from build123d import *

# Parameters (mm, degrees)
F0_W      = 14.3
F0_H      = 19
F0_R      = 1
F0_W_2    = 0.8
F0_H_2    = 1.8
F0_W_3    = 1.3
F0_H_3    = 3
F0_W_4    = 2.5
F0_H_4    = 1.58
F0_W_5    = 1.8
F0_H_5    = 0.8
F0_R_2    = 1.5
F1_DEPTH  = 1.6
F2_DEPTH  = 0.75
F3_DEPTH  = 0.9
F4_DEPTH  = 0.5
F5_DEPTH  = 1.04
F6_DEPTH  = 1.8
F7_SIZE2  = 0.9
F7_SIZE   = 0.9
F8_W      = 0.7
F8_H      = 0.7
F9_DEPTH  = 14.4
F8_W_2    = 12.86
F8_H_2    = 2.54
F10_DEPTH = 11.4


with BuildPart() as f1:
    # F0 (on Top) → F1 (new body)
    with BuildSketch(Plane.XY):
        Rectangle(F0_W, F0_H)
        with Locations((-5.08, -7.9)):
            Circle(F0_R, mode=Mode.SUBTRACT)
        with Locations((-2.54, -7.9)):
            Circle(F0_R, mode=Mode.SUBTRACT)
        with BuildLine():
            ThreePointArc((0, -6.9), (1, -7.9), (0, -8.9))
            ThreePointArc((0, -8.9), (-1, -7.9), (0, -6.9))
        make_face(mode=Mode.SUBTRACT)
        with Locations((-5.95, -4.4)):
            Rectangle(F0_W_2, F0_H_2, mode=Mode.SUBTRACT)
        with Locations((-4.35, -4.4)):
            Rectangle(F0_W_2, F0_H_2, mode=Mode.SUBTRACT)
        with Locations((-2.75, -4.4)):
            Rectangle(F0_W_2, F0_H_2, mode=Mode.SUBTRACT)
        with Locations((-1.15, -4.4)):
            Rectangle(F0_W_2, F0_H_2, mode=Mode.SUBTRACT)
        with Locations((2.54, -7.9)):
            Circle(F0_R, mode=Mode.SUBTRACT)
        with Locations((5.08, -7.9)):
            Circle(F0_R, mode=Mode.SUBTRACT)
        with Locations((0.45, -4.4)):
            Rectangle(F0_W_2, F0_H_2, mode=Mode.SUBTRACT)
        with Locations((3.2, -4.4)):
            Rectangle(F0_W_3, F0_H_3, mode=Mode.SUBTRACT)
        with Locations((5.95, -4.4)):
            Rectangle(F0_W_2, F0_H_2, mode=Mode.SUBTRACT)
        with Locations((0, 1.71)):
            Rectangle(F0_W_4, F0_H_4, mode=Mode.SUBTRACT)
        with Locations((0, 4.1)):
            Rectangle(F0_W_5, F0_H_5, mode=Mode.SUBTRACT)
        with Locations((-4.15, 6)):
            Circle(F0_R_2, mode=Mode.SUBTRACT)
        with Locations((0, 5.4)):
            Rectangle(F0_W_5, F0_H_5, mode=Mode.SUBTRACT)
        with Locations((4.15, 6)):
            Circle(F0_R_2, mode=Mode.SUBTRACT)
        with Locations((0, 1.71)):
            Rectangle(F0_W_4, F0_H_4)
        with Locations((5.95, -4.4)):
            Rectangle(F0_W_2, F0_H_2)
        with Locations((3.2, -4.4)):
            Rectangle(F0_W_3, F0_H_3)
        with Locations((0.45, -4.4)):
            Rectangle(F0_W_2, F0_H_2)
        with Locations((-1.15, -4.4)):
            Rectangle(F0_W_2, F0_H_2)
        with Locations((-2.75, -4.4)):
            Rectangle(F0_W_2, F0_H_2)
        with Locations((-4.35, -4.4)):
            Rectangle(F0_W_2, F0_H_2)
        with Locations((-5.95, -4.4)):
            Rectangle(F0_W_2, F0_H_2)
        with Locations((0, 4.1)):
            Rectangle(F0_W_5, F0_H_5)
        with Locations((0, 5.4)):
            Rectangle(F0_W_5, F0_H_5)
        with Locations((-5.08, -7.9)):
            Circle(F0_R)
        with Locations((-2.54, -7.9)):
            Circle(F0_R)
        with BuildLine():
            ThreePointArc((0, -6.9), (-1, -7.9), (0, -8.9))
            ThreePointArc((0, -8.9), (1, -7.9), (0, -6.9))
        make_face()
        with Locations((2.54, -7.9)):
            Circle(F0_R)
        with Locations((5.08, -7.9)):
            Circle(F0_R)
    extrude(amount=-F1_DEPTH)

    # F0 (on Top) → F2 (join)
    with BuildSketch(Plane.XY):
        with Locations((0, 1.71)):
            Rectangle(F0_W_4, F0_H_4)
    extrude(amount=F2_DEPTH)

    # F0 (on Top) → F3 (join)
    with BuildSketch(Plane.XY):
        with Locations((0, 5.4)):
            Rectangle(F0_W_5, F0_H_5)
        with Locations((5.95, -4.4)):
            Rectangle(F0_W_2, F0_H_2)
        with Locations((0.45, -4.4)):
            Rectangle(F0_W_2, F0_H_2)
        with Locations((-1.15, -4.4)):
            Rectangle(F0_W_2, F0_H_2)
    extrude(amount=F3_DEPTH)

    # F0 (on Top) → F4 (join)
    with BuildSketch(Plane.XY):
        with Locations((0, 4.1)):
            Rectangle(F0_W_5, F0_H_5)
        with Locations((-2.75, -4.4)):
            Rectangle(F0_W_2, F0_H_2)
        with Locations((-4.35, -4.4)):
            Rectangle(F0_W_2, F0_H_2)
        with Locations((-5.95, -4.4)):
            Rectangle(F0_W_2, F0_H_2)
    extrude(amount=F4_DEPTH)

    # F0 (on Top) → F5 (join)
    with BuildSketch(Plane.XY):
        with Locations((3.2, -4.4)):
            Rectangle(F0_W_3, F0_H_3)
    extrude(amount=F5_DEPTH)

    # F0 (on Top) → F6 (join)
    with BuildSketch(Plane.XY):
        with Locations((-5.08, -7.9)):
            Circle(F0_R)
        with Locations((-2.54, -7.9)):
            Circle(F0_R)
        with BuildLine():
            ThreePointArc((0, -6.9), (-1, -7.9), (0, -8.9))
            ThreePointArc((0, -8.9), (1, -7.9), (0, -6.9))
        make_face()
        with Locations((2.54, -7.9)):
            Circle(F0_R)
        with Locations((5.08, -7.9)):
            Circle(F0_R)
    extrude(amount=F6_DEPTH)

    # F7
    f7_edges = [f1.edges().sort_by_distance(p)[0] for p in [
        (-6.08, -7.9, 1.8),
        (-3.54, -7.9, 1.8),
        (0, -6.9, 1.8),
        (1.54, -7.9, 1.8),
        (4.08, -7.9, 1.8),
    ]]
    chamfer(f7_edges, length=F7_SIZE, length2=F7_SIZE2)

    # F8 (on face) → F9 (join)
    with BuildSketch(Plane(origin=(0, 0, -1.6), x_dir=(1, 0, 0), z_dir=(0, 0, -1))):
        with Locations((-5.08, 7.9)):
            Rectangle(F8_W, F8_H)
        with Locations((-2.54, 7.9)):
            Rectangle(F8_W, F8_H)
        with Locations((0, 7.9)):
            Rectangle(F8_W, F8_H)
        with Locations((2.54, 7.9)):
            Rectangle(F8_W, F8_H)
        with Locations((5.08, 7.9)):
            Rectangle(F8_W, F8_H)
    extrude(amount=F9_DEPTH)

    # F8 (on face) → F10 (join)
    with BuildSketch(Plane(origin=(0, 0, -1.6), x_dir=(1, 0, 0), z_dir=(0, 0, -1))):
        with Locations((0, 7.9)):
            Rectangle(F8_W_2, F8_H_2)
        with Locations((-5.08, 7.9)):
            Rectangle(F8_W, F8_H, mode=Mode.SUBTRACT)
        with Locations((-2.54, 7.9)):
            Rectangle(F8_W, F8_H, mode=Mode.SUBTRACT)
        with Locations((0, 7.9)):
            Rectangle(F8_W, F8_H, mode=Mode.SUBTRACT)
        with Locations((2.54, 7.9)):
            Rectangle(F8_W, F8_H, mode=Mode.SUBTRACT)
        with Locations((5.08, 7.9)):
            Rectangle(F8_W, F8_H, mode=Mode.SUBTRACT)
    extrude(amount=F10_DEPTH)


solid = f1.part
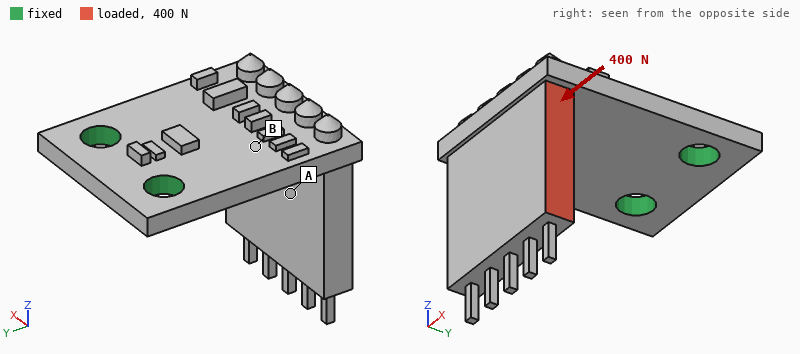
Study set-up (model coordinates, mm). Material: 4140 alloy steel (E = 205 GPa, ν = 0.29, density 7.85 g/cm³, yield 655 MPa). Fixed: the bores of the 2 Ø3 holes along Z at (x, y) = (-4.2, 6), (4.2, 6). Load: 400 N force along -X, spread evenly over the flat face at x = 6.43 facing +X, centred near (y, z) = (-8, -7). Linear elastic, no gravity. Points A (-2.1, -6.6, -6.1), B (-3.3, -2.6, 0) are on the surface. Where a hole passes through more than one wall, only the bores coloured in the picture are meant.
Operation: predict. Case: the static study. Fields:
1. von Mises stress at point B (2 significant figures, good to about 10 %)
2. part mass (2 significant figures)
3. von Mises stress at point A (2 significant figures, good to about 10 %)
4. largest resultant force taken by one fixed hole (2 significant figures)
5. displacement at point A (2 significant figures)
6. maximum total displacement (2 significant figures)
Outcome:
220 MPa
6.5 g
49 MPa
620 N
0.075 mm
0.20 mm
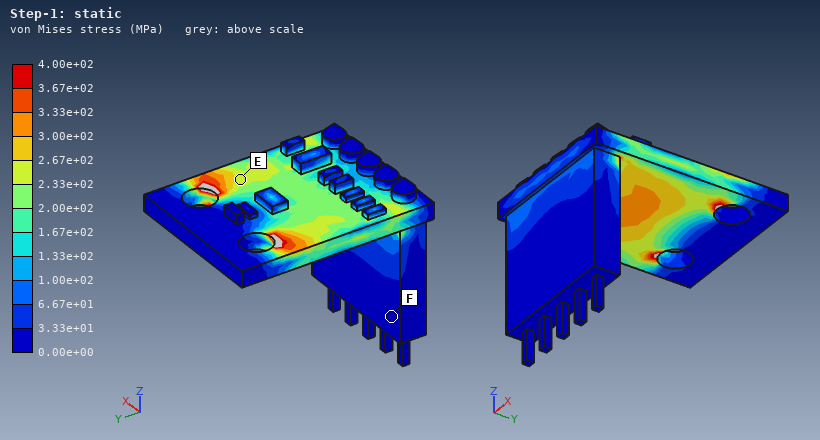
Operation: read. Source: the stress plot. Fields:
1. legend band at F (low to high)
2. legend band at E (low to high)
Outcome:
0.00e+00 to 3.33e+01 MPa
2.33e+02 to 2.67e+02 MPa
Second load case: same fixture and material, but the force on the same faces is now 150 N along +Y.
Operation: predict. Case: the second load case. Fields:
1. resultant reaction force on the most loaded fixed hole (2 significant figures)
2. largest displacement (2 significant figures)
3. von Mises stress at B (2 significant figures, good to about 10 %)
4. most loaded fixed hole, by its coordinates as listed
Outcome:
180 N
0.20 mm
140 MPa
(4.2, 6)
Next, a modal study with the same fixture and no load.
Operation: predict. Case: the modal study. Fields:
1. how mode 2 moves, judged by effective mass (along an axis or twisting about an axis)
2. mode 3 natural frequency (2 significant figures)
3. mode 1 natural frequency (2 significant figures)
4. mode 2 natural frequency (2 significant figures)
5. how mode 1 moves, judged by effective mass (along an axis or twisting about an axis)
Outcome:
along X
8300 Hz
2400 Hz
4800 Hz
along Z
